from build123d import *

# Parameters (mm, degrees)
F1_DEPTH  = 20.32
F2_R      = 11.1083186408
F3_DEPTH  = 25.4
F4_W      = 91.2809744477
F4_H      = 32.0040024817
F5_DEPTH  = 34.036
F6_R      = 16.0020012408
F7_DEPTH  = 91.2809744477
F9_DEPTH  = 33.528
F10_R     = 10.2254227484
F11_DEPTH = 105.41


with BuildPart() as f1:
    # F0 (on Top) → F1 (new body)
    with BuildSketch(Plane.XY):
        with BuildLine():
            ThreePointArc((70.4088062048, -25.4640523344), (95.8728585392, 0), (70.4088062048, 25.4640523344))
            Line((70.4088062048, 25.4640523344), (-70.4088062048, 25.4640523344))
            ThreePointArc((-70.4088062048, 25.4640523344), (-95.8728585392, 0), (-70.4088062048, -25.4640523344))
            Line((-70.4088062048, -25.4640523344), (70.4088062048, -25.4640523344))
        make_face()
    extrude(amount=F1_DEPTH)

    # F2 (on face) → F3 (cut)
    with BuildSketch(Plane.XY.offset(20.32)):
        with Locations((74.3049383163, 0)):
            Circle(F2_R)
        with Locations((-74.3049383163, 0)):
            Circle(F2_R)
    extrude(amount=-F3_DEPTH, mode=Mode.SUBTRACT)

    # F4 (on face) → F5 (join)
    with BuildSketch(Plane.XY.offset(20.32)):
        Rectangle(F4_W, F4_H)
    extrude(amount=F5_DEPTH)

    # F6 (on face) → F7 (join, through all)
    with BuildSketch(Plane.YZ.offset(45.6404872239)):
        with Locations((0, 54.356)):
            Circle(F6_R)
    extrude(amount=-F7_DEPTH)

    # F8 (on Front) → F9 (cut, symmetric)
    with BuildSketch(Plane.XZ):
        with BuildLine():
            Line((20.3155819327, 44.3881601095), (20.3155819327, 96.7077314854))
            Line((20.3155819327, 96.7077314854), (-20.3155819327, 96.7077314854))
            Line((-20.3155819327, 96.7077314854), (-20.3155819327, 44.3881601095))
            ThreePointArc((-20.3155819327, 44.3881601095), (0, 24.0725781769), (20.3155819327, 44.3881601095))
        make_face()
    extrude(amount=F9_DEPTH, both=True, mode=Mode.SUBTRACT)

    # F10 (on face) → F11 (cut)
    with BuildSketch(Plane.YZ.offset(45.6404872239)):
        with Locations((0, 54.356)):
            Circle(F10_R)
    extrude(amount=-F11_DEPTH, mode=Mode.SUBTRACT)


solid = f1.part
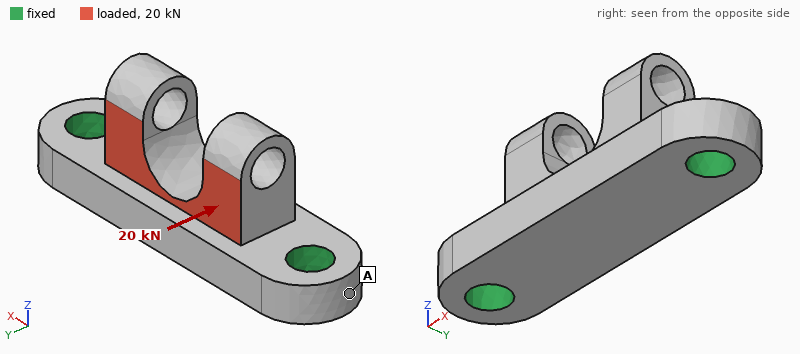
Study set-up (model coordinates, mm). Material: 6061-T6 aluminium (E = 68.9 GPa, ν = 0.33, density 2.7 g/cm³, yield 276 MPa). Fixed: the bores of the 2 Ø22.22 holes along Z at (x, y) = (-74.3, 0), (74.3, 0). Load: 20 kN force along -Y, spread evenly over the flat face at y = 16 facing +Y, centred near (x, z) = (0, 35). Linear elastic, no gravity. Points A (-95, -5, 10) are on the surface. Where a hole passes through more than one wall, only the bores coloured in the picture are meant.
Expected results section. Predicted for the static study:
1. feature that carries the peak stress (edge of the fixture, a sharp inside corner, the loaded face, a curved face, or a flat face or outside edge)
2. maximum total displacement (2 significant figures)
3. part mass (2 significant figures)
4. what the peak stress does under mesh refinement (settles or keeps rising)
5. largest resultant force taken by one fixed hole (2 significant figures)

edge of the fixture
0.19 mm
650 g
keeps rising
10 kN
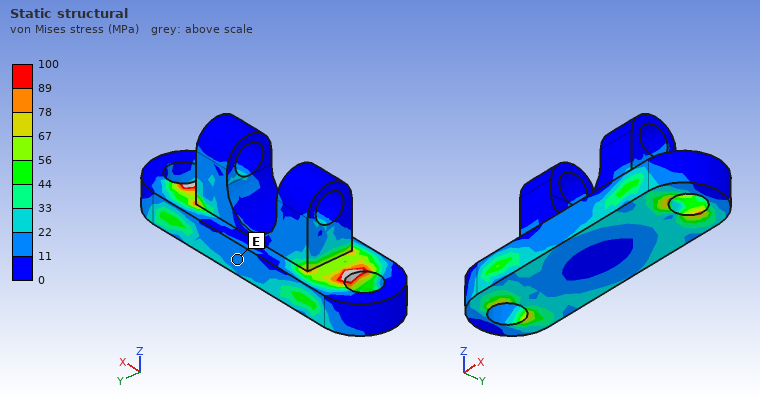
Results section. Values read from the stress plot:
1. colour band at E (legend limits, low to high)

11 to 22 MPa
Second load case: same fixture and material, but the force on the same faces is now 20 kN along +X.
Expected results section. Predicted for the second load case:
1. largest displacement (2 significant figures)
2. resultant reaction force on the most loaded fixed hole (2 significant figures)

52 µm
11 kN
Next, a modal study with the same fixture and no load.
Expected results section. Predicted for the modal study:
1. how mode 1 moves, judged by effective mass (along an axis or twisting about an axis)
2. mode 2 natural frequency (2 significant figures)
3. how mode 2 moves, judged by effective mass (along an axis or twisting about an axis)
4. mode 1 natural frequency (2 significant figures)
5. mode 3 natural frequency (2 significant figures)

along Y
4300 Hz
along Z
4000 Hz
6400 Hz
